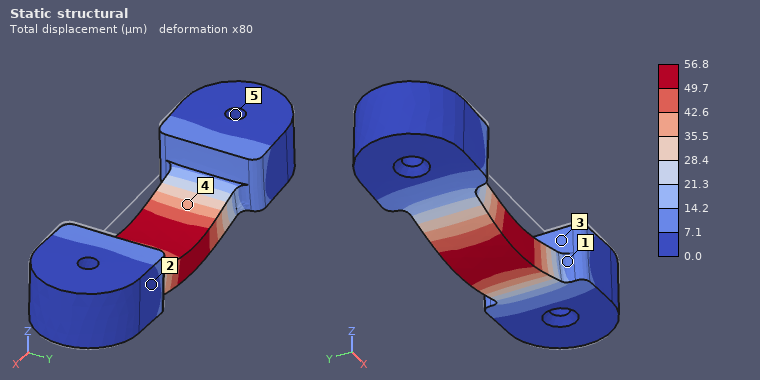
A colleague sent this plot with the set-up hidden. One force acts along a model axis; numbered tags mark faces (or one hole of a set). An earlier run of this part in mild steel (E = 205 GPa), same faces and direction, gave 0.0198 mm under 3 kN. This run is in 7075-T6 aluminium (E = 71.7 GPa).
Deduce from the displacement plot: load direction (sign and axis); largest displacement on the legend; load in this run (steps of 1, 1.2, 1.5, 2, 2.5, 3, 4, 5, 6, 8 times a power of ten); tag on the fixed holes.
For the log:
-Z
56.8 µm
3 kN
5
